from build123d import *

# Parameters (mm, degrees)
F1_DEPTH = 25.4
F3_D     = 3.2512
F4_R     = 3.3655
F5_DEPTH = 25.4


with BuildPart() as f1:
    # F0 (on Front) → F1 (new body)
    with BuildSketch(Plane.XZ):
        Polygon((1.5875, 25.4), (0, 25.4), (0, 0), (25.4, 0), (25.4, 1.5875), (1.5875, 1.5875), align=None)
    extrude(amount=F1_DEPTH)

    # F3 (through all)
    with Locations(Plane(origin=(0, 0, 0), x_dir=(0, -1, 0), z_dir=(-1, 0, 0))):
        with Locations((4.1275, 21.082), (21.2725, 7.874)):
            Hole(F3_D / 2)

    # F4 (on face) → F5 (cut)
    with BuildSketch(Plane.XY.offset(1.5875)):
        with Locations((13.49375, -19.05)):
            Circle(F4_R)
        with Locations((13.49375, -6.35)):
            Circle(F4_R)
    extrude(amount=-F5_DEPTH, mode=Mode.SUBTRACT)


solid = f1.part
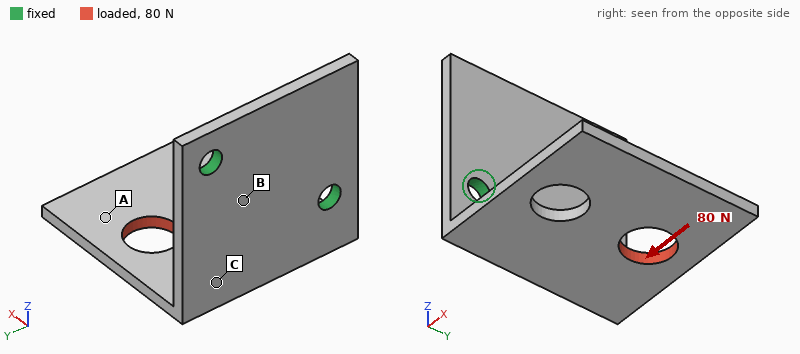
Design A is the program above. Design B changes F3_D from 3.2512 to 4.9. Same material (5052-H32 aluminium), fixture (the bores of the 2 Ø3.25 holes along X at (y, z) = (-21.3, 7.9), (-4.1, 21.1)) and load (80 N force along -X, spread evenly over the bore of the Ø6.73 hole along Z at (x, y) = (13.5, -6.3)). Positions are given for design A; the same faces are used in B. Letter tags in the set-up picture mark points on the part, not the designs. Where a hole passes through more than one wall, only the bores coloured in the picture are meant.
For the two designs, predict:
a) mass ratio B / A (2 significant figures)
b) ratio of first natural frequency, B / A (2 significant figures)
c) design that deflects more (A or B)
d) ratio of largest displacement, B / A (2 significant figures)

0.98
1.1
A
0.80
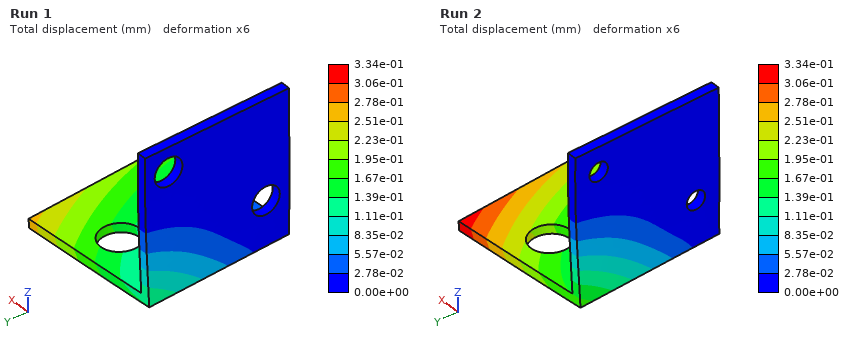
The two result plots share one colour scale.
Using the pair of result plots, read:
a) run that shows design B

Run 1
